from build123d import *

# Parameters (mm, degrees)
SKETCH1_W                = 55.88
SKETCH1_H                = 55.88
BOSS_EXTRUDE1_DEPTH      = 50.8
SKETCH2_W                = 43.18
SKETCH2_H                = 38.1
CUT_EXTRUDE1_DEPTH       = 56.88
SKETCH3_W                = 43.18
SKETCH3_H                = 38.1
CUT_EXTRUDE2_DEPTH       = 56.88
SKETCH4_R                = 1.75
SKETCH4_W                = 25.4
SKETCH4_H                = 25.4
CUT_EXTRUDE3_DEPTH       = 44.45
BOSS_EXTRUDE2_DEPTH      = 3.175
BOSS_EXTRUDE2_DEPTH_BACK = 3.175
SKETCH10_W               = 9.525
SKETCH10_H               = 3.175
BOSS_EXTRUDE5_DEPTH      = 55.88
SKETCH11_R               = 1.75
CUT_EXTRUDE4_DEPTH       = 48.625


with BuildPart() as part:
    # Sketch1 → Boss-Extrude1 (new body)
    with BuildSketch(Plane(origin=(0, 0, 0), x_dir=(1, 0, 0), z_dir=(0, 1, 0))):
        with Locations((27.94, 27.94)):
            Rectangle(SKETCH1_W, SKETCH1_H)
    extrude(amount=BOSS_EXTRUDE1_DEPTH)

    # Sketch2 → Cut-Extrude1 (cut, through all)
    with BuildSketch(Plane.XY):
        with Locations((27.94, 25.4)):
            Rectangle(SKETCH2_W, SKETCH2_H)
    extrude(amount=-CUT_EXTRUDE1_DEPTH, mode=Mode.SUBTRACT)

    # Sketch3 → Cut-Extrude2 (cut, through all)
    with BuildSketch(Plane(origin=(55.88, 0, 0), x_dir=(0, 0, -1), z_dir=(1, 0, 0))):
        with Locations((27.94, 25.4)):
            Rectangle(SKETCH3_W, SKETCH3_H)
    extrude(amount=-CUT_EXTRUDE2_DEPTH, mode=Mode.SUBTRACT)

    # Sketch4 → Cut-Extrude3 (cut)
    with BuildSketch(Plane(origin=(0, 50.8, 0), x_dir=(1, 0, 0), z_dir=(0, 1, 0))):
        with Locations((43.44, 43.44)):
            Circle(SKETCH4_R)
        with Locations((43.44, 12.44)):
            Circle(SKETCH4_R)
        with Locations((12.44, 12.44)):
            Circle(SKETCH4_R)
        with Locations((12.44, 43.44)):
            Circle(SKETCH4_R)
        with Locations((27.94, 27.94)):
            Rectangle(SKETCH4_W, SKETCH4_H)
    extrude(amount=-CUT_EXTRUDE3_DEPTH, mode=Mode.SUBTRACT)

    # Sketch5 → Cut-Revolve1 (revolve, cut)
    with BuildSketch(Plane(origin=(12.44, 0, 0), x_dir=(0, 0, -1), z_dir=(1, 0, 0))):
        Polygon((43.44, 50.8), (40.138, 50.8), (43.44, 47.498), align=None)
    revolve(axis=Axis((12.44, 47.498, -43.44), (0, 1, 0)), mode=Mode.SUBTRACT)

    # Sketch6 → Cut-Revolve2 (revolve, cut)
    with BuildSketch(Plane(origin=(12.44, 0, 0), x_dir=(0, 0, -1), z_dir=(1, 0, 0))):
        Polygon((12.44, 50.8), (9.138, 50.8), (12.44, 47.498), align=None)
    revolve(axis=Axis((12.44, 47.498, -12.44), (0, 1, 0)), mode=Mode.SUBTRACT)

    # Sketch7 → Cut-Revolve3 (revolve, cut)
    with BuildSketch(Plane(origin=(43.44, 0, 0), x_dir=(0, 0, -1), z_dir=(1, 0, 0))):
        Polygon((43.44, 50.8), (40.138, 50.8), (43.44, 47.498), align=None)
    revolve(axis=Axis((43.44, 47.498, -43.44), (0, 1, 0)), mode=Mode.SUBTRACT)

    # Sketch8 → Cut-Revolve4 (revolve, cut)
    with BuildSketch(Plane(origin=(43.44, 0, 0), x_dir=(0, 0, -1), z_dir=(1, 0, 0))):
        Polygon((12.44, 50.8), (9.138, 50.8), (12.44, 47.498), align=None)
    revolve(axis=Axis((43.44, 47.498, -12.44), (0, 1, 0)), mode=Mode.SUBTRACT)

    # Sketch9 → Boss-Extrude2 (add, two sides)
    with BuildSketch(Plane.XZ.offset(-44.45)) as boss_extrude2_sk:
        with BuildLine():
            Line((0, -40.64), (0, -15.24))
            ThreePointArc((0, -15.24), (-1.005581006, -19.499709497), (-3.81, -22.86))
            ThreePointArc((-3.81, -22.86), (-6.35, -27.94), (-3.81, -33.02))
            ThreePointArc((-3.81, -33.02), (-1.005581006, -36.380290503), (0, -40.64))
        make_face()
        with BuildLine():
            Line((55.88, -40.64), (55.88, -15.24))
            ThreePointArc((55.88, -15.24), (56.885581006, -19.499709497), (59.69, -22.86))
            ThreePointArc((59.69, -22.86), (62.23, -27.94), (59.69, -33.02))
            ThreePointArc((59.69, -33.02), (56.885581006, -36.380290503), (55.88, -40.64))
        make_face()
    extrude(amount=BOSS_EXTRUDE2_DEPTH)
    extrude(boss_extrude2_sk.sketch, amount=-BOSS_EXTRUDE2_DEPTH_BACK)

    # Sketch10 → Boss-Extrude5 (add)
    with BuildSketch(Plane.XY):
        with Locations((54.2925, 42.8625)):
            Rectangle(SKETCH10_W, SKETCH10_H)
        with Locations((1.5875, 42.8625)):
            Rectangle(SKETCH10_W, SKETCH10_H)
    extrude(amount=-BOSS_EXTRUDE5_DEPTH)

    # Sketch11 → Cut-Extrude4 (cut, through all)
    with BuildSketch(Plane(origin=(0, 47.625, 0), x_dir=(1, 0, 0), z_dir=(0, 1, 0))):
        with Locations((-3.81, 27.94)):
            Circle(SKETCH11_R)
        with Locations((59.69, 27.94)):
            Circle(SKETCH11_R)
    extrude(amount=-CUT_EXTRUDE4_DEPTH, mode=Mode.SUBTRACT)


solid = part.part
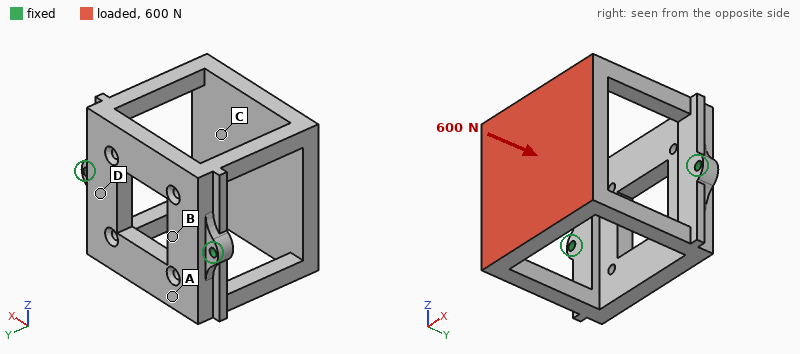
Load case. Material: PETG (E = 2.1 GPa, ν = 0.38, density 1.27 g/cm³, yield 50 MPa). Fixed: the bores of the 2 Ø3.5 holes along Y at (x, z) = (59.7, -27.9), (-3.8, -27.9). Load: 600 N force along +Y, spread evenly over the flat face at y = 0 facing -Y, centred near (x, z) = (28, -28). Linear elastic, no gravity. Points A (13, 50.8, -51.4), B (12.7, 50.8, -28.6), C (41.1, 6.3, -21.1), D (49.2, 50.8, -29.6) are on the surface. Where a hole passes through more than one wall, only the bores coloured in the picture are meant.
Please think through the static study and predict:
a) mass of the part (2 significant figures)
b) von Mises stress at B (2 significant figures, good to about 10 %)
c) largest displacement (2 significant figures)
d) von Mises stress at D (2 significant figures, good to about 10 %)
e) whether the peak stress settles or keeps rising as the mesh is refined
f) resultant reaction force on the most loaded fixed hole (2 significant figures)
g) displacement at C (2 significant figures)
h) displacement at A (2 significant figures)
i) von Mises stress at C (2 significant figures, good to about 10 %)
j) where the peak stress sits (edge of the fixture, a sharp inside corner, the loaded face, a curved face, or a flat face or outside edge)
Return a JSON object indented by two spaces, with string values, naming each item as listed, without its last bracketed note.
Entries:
{
  "mass of the part": "57 g",
  "von Mises stress at B": "12 MPa",
  "largest displacement": "0.94 mm",
  "von Mises stress at D": "14 MPa",
  "whether the peak stress settles or keeps rising as the mesh is refined": "keeps rising",
  "resultant reaction force on the most loaded fixed hole": "340 N",
  "displacement at C": "0.87 mm",
  "displacement at A": "0.40 mm",
  "von Mises stress at C": "6.2 MPa",
  "where the peak stress sits": "edge of the fixture"
}
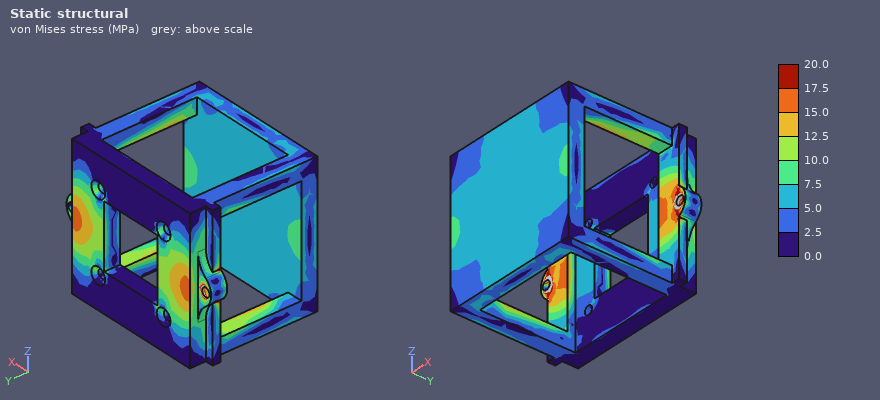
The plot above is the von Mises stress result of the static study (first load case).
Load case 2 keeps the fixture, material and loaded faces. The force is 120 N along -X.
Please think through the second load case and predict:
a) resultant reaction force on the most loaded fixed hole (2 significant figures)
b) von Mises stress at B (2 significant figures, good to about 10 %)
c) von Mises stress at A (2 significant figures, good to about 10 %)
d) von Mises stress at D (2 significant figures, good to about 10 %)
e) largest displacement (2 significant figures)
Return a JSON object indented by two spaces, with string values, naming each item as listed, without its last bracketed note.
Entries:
{
  "resultant reaction force on the most loaded fixed hole": "110 N",
  "von Mises stress at B": "2.0 MPa",
  "von Mises stress at A": "2.9 MPa",
  "von Mises stress at D": "3.7 MPa",
  "largest displacement": "1.2 mm"
}
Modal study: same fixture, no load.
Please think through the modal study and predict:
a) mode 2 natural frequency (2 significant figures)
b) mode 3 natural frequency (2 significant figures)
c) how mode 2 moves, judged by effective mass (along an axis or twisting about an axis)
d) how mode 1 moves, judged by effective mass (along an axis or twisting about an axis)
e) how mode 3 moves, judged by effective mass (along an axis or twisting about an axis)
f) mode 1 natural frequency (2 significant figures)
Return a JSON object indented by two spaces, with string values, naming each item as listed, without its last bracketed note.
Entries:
{
  "mode 2 natural frequency": "320 Hz",
  "mode 3 natural frequency": "540 Hz",
  "how mode 2 moves, judged by effective mass": "along X",
  "how mode 1 moves, judged by effective mass": "along Z",
  "how mode 3 moves, judged by effective mass": "twisting about Y",
  "mode 1 natural frequency": "220 Hz"
}
